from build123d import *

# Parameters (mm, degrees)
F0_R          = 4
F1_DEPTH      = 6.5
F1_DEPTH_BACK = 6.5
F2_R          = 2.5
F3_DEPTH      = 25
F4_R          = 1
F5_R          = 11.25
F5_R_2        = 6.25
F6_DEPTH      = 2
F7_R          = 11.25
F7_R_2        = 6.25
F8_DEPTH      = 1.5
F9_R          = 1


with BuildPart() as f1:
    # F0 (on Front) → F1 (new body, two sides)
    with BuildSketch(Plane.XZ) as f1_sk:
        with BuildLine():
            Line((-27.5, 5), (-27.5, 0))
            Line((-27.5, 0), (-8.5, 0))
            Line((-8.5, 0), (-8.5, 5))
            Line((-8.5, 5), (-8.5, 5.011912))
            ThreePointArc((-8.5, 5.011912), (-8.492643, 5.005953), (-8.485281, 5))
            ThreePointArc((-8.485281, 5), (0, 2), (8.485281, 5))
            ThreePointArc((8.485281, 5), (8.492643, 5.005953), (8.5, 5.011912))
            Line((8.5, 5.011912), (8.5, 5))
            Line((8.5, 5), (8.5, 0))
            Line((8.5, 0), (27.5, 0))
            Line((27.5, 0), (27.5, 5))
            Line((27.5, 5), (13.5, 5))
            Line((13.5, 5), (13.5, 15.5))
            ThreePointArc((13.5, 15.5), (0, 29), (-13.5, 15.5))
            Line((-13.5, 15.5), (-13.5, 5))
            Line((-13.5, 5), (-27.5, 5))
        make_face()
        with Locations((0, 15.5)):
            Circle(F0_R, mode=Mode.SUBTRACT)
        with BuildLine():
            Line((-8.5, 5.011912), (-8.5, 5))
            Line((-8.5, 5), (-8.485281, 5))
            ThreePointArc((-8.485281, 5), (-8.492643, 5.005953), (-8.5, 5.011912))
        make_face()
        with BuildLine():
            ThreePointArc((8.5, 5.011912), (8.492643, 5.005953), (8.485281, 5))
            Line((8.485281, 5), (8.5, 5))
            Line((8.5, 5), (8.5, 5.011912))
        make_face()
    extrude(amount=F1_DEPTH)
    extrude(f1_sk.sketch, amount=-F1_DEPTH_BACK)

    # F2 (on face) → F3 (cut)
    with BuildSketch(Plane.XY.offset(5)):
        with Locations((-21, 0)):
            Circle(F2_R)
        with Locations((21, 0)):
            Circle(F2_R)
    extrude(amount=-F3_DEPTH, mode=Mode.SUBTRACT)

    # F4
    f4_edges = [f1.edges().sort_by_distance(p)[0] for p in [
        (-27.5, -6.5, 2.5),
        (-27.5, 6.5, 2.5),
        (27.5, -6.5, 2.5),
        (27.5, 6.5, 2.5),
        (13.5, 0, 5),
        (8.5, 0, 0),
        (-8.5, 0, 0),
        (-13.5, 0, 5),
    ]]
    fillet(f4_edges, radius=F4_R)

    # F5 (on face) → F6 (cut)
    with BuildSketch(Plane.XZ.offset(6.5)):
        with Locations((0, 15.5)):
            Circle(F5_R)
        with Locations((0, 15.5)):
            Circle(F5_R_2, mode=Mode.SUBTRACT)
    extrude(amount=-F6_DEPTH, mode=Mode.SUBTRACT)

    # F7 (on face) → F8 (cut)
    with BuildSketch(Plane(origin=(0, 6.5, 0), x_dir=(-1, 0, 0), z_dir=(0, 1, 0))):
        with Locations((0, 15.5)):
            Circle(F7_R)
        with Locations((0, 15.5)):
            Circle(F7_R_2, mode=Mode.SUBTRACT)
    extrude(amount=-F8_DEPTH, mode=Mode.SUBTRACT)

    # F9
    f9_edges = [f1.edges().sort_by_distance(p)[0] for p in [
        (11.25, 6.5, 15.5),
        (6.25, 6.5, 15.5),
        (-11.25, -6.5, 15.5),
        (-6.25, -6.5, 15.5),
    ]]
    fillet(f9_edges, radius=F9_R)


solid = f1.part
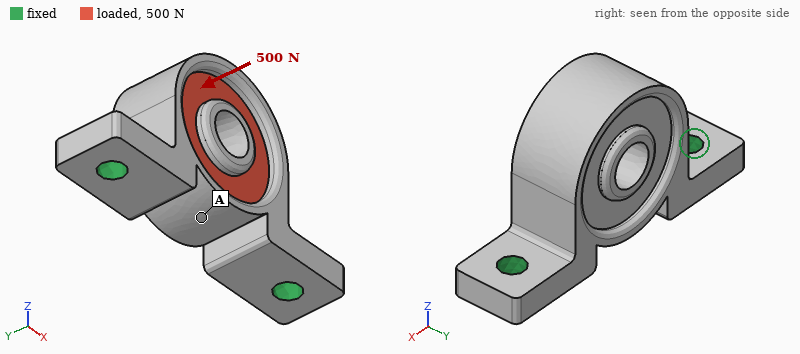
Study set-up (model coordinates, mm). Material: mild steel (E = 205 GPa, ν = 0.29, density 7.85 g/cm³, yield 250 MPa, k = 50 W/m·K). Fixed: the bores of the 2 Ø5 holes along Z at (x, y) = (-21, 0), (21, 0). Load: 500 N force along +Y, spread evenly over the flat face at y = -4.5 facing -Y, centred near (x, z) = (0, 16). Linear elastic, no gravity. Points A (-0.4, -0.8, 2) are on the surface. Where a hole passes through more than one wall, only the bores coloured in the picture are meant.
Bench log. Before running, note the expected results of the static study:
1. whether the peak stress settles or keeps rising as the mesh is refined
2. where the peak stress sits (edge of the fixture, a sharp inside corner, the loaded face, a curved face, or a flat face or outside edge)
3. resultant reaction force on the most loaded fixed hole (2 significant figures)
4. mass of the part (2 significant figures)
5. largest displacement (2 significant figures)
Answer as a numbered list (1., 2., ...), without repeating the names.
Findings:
1. keeps rising
2. edge of the fixture
3. 250 N
4. 66 g
5. 20 µm
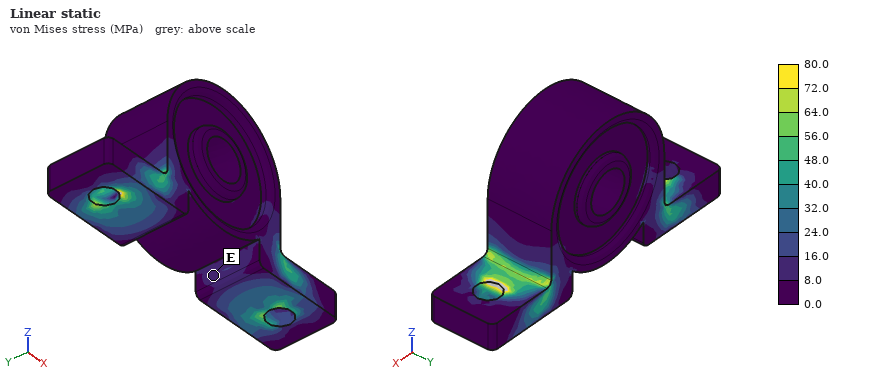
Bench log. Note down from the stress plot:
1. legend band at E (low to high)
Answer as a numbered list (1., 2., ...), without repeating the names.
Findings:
1. 8.0 to 16.0 MPa
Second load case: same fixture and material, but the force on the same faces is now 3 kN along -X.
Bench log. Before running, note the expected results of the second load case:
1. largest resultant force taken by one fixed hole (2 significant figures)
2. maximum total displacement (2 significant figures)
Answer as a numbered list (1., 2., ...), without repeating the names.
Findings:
1. 1.9 kN
2. 14 µm
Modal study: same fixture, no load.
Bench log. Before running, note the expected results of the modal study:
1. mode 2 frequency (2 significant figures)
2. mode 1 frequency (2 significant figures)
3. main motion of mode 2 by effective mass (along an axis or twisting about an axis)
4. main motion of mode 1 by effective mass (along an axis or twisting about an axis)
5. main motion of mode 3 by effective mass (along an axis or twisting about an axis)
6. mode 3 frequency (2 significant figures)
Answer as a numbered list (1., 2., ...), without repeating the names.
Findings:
1. 14 kHz
2. 4600 Hz
3. along X
4. along Y
5. along Z
6. 14 kHz
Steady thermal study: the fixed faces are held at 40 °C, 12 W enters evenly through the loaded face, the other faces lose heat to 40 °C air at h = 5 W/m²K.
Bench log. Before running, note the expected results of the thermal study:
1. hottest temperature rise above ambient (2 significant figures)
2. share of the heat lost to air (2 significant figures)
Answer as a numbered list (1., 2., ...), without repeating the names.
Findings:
1. 32 K
2. 3.1 %
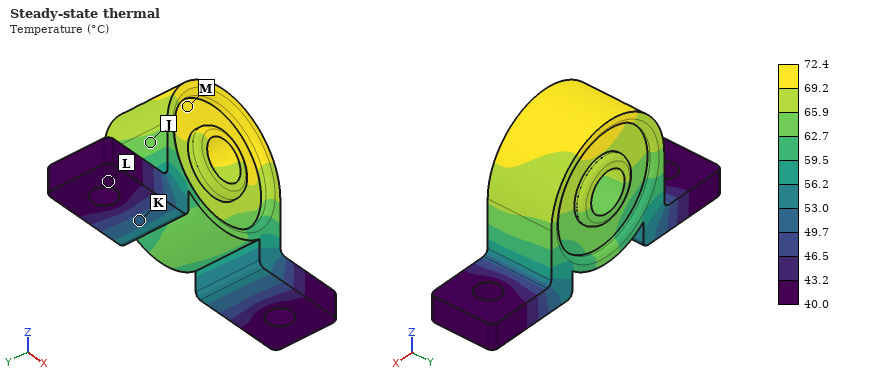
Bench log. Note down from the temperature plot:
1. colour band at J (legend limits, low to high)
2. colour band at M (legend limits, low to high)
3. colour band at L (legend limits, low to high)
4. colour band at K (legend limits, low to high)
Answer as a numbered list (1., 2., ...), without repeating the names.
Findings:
1. 62.7 to 65.9 °C
2. 69.2 to 72.4 °C
3. 40.0 to 43.2 °C
4. 49.7 to 53.0 °C
